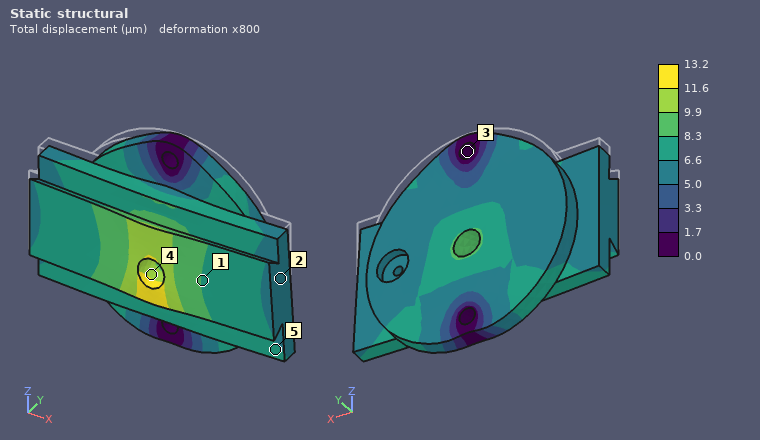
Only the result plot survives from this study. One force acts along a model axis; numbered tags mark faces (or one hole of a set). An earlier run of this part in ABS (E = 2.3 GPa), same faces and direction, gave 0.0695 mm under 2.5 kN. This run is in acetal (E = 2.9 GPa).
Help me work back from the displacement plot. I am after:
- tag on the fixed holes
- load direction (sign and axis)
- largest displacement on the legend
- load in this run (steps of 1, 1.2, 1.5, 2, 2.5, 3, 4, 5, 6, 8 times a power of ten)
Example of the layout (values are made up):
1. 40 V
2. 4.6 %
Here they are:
1. 3
2. -Z
3. 13.2 µm
4. 600 N
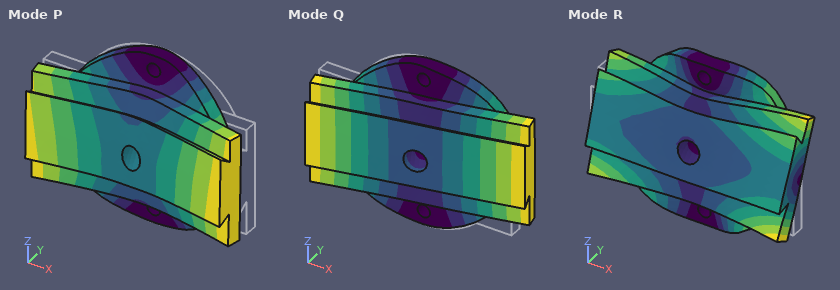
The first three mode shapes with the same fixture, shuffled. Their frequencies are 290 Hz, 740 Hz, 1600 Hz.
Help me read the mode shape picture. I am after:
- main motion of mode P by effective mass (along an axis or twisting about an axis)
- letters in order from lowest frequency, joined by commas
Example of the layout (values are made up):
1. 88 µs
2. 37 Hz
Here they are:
1. along Y
2. Q, P, R
